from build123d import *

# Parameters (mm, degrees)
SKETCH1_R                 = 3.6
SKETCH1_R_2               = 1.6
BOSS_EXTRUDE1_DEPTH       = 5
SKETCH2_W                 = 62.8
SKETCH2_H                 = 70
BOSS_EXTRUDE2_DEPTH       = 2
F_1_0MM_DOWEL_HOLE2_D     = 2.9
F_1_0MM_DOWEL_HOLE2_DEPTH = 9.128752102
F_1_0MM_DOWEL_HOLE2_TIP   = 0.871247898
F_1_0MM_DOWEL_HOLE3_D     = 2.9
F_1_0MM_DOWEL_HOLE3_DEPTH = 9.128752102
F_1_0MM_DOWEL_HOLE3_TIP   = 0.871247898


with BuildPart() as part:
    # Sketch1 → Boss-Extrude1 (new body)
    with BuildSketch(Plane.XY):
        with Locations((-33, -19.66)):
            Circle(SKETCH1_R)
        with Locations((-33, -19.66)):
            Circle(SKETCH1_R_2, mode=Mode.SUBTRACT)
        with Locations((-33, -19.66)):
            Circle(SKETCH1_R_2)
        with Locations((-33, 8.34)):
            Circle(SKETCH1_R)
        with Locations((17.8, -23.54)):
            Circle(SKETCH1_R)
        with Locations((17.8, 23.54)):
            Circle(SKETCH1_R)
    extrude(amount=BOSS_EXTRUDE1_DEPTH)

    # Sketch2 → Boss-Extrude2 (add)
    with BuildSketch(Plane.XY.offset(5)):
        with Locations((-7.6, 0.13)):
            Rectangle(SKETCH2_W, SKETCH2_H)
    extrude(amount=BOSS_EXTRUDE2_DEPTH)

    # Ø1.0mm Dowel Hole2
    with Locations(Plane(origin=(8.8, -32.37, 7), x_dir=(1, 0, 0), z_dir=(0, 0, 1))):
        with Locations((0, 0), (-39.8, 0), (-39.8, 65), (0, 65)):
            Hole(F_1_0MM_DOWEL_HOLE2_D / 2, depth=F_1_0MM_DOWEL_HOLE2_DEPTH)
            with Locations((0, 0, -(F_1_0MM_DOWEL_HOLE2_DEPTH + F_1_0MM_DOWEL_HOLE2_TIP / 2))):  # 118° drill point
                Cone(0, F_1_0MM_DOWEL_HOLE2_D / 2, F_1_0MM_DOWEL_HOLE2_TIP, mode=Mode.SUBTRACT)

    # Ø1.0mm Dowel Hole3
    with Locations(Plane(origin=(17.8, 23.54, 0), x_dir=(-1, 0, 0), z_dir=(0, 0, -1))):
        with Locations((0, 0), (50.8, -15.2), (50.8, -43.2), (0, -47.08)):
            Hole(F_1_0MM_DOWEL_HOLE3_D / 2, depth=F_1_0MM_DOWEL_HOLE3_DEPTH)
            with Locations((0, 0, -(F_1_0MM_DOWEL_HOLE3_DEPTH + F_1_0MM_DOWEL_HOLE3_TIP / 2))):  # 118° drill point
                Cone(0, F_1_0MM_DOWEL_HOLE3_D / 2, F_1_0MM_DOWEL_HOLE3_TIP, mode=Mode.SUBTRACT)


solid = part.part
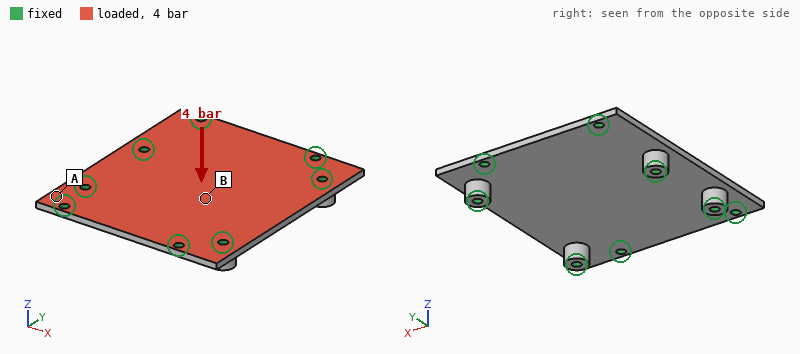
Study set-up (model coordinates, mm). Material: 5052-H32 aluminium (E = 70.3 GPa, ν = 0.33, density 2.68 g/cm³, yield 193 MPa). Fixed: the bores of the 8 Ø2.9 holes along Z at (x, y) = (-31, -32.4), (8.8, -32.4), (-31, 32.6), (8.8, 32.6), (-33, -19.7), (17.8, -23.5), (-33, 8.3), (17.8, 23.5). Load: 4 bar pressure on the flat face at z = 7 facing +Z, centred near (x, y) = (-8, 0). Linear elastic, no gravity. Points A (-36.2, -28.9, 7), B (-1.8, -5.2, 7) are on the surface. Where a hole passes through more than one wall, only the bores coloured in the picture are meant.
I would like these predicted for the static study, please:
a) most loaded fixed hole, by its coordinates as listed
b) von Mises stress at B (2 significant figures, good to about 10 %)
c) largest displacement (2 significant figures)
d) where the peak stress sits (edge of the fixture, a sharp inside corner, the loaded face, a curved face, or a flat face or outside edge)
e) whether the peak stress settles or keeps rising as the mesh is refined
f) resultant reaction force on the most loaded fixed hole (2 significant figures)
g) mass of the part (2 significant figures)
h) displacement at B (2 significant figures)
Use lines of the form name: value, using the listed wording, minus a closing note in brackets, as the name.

most loaded fixed hole, by its coordinates as listed: (-33, 8.3)
von Mises stress at B: 55 MPa
largest displacement: 0.18 mm
where the peak stress sits: edge of the fixture
whether the peak stress settles or keeps rising as the mesh is refined: keeps rising
resultant reaction force on the most loaded fixed hole: 360 N
mass of the part: 25 g
displacement at B: 0.17 mm
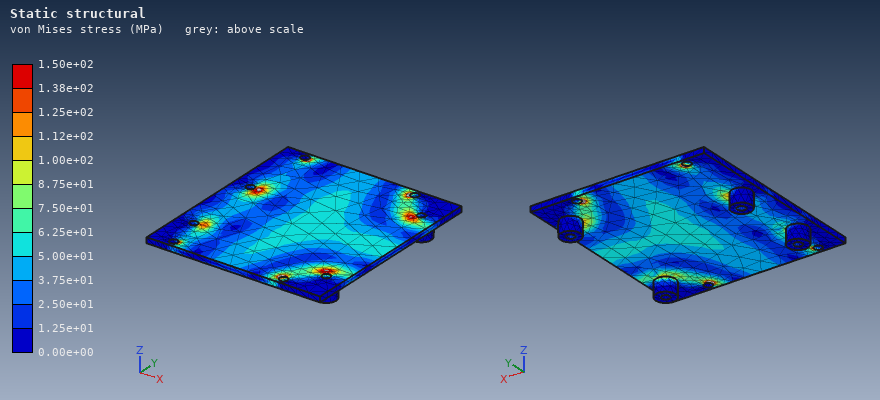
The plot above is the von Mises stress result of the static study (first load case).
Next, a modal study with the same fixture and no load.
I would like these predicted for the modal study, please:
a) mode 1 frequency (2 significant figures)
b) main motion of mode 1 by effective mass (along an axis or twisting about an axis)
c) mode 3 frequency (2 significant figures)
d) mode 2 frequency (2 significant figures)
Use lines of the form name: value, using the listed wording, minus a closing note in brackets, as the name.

mode 1 frequency: 4100 Hz
main motion of mode 1 by effective mass: along Z
mode 3 frequency: 6400 Hz
mode 2 frequency: 6300 Hz
